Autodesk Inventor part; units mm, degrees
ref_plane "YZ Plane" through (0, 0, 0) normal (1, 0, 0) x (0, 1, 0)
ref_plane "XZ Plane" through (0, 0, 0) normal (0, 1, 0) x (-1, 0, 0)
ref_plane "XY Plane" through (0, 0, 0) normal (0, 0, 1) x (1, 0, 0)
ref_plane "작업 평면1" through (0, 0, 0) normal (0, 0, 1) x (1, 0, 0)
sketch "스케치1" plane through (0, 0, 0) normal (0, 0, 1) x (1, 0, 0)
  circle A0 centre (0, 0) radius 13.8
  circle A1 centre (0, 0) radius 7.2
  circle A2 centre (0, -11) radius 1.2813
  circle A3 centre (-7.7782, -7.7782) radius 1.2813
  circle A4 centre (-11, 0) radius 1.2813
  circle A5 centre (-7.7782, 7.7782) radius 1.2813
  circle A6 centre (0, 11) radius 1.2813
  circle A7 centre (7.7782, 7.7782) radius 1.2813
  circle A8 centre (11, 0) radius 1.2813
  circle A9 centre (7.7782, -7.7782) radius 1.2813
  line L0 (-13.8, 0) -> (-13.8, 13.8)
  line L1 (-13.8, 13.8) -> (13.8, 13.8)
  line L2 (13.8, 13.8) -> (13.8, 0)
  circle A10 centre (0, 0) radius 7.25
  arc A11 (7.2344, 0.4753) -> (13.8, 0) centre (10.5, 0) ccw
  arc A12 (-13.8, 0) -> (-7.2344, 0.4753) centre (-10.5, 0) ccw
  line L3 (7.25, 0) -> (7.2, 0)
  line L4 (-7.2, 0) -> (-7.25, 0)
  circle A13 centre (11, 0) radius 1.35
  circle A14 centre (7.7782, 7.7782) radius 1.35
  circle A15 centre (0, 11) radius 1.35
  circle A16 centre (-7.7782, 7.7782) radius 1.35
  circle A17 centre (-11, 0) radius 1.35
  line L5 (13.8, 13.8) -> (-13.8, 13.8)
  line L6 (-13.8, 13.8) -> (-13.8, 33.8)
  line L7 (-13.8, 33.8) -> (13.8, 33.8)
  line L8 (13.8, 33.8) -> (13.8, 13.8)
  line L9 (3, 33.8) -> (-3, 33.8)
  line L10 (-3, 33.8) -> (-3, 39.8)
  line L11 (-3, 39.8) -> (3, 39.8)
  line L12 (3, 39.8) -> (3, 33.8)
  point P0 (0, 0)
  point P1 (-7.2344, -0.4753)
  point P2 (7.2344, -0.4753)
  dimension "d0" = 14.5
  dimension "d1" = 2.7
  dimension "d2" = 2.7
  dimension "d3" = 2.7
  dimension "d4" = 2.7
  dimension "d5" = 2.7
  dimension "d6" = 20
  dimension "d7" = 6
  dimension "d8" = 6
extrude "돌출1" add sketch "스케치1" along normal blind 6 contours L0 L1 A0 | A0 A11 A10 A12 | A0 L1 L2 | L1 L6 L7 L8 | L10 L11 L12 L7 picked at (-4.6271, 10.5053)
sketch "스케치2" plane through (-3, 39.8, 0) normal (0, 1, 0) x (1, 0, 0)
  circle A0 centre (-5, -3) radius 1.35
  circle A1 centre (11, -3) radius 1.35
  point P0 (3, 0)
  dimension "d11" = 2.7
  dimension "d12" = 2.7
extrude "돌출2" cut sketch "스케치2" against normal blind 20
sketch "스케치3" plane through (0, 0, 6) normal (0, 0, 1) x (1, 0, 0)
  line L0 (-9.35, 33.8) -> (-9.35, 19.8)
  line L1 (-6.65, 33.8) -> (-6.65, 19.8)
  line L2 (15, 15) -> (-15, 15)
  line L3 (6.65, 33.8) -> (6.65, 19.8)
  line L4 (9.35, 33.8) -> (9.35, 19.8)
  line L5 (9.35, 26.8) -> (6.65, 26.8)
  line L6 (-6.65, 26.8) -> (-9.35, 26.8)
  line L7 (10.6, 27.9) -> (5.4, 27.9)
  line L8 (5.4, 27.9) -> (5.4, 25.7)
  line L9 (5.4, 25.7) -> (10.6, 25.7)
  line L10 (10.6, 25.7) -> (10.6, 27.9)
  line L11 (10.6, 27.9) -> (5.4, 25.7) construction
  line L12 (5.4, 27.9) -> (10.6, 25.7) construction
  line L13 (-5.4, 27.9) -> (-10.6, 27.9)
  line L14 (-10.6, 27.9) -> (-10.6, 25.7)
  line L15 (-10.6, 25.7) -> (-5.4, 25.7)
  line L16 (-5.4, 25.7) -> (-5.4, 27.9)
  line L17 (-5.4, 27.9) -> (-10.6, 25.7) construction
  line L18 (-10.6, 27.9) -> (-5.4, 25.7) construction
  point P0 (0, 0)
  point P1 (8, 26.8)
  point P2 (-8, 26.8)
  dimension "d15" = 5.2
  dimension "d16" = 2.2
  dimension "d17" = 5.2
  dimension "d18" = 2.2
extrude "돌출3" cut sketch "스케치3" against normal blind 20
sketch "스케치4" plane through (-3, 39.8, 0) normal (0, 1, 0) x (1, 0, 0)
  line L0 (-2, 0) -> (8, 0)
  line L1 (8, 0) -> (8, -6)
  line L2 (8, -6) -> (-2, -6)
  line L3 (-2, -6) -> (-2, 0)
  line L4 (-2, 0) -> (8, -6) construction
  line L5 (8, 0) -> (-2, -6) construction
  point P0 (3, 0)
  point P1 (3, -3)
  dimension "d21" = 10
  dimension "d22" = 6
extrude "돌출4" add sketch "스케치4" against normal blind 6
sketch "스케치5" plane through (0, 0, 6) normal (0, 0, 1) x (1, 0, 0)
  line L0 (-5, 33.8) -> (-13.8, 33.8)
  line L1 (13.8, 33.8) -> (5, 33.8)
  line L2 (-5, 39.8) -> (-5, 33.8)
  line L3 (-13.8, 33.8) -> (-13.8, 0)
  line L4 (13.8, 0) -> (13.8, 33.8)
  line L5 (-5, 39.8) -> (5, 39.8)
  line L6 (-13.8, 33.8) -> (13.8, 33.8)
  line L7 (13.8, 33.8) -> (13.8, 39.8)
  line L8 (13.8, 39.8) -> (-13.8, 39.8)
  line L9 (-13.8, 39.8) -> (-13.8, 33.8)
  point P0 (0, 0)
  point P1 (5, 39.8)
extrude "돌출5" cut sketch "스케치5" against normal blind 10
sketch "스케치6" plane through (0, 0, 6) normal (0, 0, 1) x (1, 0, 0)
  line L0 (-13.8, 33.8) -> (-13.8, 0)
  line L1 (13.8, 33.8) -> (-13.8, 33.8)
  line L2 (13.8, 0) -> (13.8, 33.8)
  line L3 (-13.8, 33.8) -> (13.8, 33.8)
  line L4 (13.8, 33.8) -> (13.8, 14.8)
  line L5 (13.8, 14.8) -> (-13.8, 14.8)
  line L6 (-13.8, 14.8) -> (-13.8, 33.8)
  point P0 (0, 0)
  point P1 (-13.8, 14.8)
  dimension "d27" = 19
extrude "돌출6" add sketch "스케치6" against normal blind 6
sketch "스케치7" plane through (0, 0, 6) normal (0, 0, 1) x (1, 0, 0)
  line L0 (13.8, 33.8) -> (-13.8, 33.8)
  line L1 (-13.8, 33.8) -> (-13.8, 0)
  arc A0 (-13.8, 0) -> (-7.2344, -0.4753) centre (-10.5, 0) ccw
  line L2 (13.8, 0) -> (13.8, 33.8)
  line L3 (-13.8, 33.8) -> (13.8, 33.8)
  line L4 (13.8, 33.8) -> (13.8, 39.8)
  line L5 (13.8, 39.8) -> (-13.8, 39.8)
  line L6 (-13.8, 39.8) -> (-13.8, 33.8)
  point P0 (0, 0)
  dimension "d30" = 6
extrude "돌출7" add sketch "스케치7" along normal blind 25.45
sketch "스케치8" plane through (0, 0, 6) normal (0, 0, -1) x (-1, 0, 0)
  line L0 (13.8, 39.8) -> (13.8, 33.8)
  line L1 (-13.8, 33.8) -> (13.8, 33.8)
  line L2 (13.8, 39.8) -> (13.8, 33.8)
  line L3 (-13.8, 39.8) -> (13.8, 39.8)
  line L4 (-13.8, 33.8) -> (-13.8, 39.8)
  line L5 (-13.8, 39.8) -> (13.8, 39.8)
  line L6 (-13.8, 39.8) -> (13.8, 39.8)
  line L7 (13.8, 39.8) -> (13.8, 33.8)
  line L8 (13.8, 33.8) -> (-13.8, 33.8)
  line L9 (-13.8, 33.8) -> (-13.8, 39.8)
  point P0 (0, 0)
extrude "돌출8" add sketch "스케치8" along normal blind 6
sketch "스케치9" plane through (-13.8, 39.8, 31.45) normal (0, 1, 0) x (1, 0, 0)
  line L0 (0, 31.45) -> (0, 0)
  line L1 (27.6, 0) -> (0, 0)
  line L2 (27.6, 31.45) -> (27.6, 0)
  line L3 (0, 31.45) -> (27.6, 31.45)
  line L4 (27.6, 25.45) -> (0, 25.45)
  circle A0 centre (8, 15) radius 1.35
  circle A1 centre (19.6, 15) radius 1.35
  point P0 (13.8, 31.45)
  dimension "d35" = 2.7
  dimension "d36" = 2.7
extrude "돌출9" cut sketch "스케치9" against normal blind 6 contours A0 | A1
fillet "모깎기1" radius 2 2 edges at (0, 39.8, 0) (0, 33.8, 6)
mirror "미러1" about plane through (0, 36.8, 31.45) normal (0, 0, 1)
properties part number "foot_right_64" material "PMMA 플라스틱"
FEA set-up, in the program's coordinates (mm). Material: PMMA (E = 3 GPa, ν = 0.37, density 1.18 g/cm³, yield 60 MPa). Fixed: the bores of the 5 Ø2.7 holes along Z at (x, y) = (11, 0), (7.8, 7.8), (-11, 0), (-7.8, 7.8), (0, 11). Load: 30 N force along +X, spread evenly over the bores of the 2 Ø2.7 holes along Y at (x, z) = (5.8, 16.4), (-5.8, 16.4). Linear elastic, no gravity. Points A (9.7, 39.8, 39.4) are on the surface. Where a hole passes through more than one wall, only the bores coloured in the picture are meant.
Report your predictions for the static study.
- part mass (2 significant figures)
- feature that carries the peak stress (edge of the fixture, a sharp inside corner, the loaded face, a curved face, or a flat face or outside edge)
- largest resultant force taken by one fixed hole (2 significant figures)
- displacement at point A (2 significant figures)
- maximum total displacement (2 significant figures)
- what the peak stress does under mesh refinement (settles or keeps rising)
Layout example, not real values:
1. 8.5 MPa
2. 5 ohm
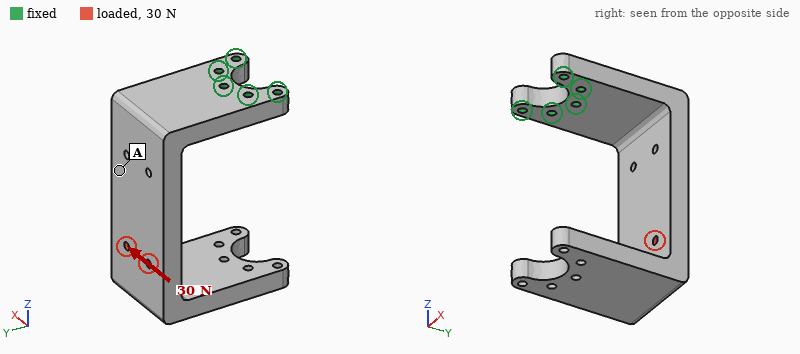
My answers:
1. 24 g
2. edge of the fixture
3. 62 N
4. 0.31 mm
5. 0.92 mm
6. keeps rising
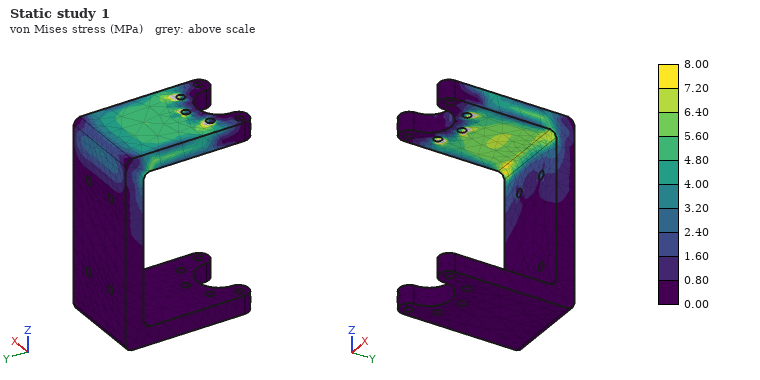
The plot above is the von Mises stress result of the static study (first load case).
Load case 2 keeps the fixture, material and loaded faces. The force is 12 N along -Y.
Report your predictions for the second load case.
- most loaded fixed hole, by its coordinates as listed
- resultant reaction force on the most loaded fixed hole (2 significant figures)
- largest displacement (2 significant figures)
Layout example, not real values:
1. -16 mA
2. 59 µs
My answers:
1. (0, 11)
2. 24 N
3. 0.95 mm
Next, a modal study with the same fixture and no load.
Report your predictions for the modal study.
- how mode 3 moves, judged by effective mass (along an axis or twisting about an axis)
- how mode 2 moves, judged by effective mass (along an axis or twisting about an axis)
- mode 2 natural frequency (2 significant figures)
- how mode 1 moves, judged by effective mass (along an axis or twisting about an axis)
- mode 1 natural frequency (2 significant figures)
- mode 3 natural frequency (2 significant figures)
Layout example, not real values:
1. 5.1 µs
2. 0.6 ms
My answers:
1. along Z
2. along X
3. 240 Hz
4. along Y
5. 160 Hz
6. 530 Hz
